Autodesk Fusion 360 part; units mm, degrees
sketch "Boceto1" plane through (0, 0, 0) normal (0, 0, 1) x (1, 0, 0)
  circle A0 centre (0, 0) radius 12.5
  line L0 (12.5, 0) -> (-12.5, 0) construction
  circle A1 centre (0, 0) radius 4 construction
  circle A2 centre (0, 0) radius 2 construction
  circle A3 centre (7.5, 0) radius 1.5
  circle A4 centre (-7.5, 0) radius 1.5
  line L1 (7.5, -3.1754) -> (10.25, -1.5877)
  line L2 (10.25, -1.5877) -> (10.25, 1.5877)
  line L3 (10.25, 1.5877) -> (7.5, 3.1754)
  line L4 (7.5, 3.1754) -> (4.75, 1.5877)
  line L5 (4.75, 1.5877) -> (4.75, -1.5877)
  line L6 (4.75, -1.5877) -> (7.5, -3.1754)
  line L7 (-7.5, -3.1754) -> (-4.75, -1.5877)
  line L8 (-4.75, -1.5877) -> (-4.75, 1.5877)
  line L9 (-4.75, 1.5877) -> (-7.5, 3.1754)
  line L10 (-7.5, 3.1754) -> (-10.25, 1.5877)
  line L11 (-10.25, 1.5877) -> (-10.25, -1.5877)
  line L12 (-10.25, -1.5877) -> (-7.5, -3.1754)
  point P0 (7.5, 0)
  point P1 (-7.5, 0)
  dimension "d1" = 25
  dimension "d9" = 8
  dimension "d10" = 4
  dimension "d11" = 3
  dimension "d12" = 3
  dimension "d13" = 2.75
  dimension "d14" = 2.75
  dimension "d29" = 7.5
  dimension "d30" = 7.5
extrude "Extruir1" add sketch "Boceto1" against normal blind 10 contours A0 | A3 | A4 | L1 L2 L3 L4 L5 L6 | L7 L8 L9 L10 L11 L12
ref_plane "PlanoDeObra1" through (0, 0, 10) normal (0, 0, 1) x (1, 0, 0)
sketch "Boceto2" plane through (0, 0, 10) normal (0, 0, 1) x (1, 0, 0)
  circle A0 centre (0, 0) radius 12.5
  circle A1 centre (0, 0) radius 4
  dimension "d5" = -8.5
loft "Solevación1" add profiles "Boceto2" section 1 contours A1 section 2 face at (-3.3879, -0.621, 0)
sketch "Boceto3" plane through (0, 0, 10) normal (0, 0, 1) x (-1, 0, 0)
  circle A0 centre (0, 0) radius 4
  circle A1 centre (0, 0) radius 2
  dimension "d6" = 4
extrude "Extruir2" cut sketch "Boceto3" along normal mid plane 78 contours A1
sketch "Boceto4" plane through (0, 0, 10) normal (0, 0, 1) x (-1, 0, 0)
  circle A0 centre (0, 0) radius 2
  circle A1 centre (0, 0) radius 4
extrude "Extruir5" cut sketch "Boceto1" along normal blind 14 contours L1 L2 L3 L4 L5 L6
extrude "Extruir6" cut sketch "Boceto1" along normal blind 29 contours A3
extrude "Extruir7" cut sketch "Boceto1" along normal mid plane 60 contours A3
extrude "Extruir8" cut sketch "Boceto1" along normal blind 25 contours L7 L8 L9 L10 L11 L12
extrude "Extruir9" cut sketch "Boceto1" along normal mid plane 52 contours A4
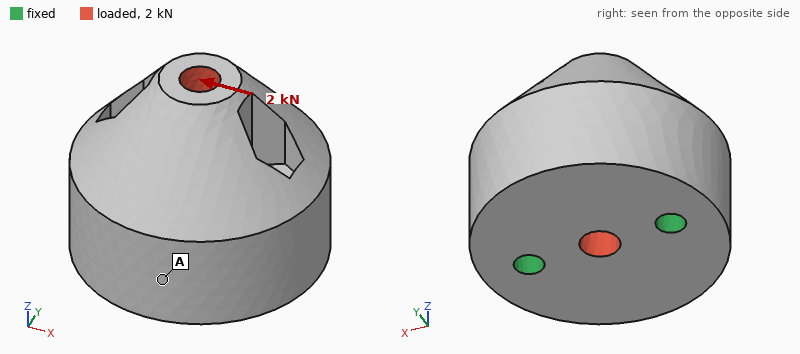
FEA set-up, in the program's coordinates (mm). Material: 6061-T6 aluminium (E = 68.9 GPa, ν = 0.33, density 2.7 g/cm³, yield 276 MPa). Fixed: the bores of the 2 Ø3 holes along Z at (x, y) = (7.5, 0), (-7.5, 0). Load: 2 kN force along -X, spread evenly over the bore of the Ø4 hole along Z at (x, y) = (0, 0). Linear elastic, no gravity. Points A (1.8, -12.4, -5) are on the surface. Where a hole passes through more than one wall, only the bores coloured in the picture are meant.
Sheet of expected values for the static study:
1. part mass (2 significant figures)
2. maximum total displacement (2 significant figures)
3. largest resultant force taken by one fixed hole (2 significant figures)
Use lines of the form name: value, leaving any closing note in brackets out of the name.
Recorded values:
part mass: 18 g
maximum total displacement: 4.3 µm
largest resultant force taken by one fixed hole: 1.1 kN
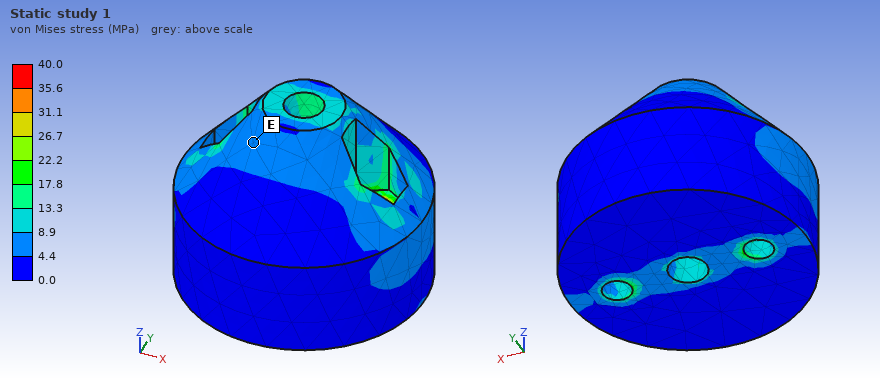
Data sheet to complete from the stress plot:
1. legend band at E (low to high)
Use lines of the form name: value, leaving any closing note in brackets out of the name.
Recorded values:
legend band at E: 4.4 to 8.9 MPa
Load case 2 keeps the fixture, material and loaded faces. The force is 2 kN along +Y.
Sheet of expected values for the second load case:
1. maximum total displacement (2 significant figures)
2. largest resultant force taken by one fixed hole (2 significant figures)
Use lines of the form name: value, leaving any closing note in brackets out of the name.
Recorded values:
maximum total displacement: 7.0 µm
largest resultant force taken by one fixed hole: 1.0 kN
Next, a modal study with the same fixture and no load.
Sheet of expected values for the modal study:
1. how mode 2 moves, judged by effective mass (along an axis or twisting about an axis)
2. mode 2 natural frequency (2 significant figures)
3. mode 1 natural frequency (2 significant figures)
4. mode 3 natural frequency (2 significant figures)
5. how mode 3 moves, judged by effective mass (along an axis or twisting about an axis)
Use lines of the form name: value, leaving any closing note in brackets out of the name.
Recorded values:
how mode 2 moves, judged by effective mass: along Z
mode 2 natural frequency: 46 kHz
mode 1 natural frequency: 28 kHz
mode 3 natural frequency: 49 kHz
how mode 3 moves, judged by effective mass: along X
